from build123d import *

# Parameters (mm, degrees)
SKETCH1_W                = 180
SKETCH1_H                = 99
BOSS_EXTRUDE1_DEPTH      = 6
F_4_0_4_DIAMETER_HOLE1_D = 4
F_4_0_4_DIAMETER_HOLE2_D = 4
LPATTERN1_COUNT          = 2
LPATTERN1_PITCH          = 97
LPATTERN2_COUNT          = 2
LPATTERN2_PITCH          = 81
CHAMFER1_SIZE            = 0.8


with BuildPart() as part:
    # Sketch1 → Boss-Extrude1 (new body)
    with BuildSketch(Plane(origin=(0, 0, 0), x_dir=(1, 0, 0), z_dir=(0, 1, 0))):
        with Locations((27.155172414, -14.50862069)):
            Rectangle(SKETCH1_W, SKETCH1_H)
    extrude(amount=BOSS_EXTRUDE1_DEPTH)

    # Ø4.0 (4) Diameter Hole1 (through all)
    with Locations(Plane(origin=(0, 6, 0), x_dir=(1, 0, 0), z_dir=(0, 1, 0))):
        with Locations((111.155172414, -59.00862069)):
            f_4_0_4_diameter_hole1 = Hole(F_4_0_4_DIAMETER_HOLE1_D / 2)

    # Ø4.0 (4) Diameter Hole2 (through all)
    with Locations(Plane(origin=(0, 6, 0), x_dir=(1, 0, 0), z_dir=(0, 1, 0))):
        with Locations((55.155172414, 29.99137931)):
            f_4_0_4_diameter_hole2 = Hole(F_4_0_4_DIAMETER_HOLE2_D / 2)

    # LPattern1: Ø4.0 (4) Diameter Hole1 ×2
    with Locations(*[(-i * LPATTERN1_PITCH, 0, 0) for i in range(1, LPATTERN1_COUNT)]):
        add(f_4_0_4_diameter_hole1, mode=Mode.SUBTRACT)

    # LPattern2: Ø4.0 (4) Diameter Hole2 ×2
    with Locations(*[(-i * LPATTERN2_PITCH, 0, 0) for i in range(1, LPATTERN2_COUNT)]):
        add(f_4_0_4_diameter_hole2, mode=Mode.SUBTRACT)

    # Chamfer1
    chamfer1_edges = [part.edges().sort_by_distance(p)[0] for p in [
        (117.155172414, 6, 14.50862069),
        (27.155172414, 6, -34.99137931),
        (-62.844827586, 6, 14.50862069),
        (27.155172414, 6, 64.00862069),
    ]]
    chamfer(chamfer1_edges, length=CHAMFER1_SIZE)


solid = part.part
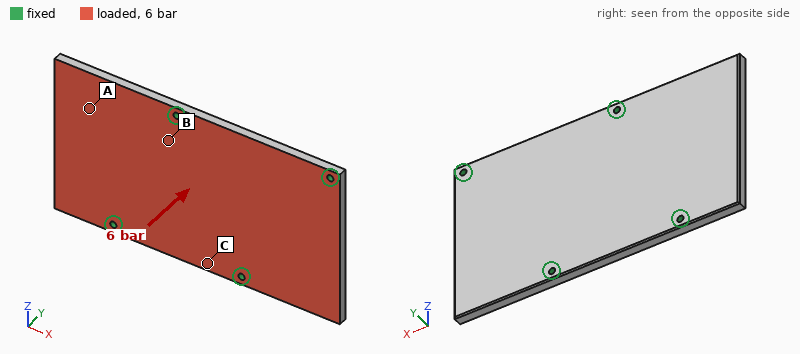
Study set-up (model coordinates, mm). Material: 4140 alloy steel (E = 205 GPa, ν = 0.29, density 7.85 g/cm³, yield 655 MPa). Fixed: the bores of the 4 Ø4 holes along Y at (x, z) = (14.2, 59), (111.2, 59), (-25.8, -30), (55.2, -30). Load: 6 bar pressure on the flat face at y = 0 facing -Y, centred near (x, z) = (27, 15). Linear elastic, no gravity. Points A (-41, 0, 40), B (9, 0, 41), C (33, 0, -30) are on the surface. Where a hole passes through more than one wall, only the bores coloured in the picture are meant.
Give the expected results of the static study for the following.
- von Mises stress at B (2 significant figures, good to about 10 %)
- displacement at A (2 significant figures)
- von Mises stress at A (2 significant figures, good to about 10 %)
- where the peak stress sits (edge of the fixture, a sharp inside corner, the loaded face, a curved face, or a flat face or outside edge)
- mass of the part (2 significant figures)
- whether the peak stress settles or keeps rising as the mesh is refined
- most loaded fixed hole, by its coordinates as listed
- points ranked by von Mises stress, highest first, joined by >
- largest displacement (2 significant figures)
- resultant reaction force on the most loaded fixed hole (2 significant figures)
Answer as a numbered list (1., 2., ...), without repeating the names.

1. 120 MPa
2. 0.29 mm
3. 60 MPa
4. edge of the fixture
5. 840 g
6. keeps rising
7. (14.2, 59)
8. B > A > C
9. 0.49 mm
10. 3.4 kN
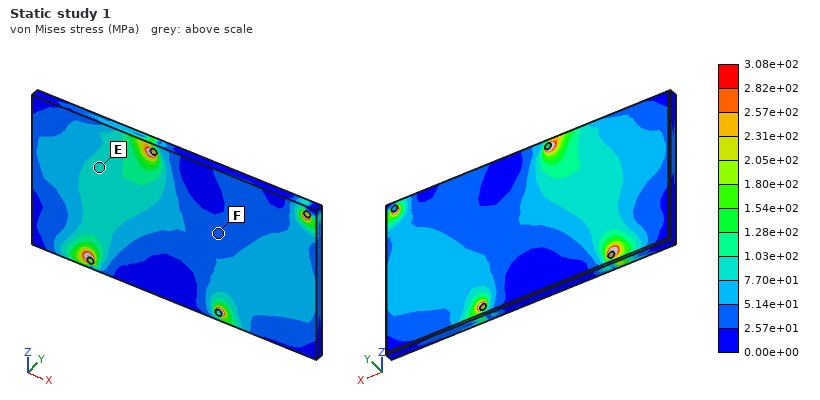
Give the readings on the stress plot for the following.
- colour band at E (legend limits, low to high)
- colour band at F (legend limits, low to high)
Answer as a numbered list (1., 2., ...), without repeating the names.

1. 7.70e+01 to 1.03e+02 MPa
2. 2.57e+01 to 5.14e+01 MPa
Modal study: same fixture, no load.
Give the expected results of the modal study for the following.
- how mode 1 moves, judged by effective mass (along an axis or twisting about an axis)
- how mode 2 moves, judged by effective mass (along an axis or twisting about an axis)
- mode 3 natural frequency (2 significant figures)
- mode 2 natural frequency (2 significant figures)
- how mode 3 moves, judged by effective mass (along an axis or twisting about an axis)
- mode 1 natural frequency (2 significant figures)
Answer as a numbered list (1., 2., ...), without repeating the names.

1. along Y
2. along Y
3. 2500 Hz
4. 1600 Hz
5. along Y
6. 1100 Hz
